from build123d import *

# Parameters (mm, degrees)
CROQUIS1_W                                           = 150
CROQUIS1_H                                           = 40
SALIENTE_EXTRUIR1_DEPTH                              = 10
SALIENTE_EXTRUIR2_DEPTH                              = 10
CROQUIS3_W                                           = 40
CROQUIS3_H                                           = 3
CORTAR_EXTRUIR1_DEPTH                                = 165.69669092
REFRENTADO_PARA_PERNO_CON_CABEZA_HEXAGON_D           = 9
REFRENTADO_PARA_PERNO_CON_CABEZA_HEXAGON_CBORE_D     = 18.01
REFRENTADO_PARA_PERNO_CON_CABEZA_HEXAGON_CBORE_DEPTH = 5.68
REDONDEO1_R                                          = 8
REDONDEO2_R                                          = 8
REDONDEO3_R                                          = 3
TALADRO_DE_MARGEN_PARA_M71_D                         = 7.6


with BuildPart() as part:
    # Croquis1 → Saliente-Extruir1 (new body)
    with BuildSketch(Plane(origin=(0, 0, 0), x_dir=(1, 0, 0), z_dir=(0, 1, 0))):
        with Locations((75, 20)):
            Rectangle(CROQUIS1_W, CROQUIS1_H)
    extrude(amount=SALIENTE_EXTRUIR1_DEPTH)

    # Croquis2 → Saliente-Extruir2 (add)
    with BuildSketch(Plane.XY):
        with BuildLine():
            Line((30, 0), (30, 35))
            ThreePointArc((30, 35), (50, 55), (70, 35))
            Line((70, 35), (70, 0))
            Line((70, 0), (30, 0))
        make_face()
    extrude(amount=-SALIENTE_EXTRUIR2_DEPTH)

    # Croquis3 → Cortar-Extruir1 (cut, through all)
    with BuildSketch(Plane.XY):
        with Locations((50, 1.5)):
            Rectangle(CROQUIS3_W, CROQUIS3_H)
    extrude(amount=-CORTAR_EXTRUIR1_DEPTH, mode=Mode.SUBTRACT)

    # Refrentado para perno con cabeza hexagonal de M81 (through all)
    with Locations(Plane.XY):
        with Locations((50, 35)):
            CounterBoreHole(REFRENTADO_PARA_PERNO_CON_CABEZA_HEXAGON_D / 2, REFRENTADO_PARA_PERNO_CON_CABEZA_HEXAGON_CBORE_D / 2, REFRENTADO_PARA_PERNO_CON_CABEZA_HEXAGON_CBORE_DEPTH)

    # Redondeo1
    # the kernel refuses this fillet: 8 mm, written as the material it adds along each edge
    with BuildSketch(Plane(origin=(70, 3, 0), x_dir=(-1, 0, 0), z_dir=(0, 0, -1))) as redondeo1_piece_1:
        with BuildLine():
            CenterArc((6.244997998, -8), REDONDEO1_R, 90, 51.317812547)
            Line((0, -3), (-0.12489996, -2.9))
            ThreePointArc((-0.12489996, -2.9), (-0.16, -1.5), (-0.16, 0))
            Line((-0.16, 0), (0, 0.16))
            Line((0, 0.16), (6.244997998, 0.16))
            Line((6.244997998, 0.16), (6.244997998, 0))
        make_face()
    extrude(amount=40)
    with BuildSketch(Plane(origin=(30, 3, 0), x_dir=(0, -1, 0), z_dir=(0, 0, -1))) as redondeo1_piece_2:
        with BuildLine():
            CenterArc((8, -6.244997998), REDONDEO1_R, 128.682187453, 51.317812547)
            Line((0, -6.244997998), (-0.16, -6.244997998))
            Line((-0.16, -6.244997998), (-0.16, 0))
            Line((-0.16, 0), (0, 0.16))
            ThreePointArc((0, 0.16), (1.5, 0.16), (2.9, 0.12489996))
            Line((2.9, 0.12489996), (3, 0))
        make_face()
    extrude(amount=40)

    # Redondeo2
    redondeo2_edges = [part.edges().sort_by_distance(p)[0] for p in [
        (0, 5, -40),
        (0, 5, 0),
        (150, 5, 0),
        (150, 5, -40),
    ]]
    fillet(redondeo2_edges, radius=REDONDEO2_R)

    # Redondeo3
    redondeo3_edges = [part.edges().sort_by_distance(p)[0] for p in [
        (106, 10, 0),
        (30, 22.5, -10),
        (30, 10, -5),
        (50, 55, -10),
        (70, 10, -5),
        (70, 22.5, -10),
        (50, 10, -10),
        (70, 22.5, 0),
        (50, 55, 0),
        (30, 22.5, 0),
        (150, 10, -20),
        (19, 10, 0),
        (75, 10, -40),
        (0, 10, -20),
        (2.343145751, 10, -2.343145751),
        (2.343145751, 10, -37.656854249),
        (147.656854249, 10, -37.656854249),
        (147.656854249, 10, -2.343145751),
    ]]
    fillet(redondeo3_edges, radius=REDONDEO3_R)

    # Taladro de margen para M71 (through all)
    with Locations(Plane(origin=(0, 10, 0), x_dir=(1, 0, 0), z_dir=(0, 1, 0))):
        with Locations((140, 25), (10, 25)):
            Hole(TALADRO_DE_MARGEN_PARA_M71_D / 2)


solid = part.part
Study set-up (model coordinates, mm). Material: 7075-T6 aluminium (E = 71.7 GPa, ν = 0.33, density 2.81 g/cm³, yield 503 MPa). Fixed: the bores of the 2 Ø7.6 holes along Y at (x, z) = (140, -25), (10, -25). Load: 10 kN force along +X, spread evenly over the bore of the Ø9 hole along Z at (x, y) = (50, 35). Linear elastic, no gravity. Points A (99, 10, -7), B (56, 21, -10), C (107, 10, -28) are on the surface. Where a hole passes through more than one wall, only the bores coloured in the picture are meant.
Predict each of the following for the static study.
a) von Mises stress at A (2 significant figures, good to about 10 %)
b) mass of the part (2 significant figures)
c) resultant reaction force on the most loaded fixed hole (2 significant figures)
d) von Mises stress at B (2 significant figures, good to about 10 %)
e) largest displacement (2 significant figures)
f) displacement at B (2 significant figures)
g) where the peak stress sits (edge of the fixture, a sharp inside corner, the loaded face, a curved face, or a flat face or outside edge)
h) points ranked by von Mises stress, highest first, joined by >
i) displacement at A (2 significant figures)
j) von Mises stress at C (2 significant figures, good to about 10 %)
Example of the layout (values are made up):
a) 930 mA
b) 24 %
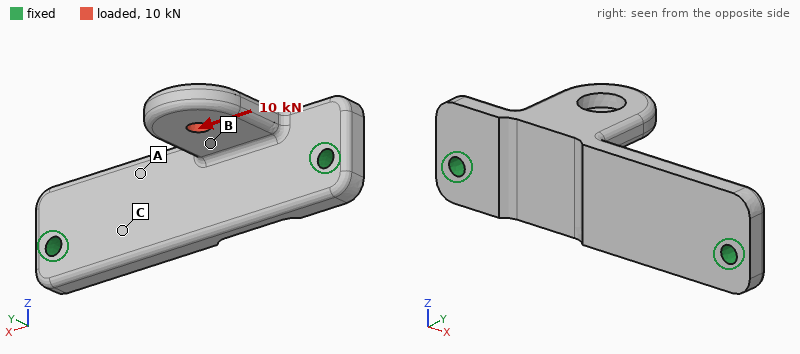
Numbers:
a) 83 MPa
b) 190 g
c) 6.1 kN
d) 120 MPa
e) 0.72 mm
f) 0.34 mm
g) a curved face
h) B > A > C
i) 0.31 mm
j) 39 MPa
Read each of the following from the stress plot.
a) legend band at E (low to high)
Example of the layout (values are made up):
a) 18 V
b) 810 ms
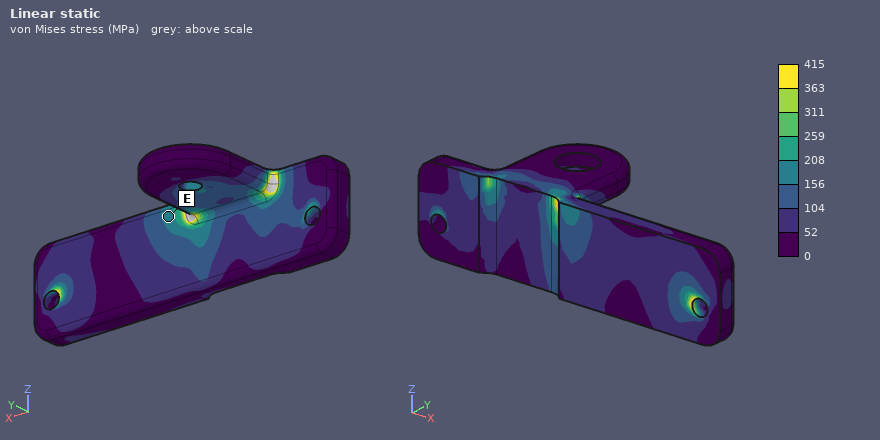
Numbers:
a) 156 to 208 MPa
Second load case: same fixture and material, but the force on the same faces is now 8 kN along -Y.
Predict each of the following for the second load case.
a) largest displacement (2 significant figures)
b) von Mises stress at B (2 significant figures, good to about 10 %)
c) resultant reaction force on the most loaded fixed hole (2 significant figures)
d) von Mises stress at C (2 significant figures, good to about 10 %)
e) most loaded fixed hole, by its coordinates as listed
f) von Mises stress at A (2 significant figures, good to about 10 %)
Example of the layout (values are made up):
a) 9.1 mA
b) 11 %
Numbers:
a) 0.59 mm
b) 52 MPa
c) 6.3 kN
d) 48 MPa
e) (10, -25)
f) 65 MPa
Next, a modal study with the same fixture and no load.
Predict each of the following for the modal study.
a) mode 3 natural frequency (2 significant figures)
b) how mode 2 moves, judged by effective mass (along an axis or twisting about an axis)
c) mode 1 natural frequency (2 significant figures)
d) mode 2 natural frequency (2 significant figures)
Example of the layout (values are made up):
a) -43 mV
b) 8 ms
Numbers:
a) 5000 Hz
b) along Y
c) 2000 Hz
d) 2500 Hz
